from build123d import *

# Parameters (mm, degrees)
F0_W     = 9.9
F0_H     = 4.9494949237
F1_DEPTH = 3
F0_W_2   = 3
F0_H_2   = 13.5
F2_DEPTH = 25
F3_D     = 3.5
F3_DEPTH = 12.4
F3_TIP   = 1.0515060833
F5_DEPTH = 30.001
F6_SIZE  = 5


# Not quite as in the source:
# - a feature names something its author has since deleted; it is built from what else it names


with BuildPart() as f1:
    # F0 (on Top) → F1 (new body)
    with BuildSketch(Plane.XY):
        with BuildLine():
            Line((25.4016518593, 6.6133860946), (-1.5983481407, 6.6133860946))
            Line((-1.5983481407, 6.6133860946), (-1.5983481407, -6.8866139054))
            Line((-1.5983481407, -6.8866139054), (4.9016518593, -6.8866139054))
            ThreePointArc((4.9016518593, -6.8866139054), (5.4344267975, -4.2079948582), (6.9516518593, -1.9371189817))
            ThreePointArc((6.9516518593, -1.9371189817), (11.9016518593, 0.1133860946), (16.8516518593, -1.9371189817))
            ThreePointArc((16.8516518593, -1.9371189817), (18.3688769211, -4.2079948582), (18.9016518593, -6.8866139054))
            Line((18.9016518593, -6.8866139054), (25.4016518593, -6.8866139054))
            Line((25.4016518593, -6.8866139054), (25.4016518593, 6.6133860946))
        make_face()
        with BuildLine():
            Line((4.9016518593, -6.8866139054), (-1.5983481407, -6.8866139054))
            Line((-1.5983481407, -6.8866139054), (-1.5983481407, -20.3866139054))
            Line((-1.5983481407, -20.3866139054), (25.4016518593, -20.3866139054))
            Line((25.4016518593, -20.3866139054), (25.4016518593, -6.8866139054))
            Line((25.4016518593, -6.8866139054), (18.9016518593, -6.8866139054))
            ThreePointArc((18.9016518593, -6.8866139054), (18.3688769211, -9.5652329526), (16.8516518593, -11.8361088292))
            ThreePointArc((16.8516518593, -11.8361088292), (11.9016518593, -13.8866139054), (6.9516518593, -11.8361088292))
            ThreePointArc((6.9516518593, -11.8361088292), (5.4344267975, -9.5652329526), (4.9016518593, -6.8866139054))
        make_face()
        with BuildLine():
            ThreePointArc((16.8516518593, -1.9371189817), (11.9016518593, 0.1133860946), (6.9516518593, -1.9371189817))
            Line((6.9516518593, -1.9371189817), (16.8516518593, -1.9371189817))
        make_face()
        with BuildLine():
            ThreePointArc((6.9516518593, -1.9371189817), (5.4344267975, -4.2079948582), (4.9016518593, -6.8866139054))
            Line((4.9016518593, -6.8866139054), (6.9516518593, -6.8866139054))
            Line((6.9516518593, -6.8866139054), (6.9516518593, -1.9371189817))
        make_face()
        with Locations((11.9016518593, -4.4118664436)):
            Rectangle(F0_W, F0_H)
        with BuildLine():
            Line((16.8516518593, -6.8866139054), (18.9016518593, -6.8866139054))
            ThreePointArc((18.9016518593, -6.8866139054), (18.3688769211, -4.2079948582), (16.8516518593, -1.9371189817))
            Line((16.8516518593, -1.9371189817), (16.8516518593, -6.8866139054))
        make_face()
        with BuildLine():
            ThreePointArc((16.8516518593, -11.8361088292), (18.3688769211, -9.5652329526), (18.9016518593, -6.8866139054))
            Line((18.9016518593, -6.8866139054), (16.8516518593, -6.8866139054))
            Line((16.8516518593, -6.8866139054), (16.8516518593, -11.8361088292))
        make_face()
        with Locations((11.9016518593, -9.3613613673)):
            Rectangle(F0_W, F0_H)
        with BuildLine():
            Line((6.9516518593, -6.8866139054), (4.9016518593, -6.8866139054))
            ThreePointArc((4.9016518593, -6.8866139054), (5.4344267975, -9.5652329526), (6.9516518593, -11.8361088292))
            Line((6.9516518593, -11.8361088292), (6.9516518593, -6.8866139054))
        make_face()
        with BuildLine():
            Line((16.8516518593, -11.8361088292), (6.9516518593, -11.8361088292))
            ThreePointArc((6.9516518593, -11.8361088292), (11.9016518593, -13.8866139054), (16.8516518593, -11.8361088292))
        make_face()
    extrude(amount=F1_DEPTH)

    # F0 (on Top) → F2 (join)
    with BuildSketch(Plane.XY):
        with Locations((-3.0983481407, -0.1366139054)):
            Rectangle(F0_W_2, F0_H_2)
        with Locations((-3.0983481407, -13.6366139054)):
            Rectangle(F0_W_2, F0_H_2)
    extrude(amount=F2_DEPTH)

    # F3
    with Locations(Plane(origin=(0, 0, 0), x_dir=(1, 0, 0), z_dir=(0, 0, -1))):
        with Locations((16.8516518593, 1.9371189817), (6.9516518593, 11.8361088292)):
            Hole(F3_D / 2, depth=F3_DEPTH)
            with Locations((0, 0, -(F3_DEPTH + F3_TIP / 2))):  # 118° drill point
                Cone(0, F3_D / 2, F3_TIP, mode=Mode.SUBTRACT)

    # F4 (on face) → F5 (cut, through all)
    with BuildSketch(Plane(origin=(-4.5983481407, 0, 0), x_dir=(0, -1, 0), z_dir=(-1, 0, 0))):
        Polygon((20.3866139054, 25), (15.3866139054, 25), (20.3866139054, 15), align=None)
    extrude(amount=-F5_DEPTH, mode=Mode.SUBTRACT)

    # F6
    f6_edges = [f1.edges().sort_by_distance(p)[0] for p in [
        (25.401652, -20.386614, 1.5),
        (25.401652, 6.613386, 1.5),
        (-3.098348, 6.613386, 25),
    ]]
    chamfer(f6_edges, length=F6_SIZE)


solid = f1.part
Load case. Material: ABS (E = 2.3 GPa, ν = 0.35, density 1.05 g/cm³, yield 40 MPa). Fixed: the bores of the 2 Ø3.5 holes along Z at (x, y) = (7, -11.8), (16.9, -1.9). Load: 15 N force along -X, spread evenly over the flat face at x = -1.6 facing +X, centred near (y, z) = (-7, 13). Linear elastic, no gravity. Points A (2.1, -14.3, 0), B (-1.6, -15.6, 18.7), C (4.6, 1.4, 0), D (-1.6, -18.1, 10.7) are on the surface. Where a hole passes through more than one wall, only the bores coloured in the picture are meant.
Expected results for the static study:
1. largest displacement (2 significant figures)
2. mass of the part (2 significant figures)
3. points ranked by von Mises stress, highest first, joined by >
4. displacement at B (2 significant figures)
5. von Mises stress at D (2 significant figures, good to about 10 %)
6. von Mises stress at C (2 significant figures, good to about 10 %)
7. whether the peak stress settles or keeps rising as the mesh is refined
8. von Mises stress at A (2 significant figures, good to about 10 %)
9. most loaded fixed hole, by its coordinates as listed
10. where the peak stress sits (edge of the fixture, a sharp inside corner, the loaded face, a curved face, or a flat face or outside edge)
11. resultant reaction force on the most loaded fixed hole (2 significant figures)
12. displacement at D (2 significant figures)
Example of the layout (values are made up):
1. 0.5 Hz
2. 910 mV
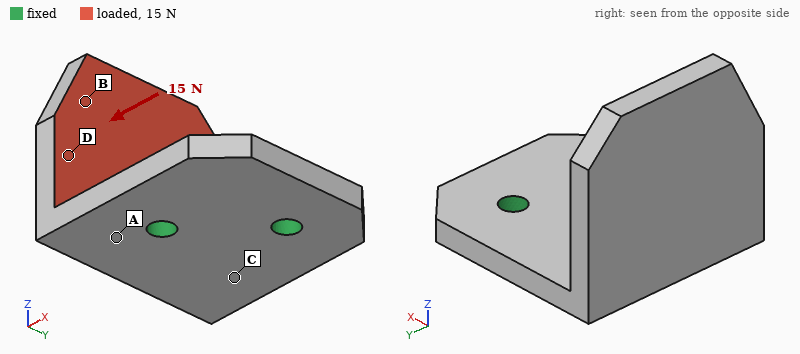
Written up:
1. 0.47 mm
2. 4.2 g
3. A > C > D > B
4. 0.31 mm
5. 1.6 MPa
6. 2.8 MPa
7. keeps rising
8. 4.4 MPa
9. (7, -11.8)
10. edge of the fixture
11. 9.9 N
12. 0.15 mm
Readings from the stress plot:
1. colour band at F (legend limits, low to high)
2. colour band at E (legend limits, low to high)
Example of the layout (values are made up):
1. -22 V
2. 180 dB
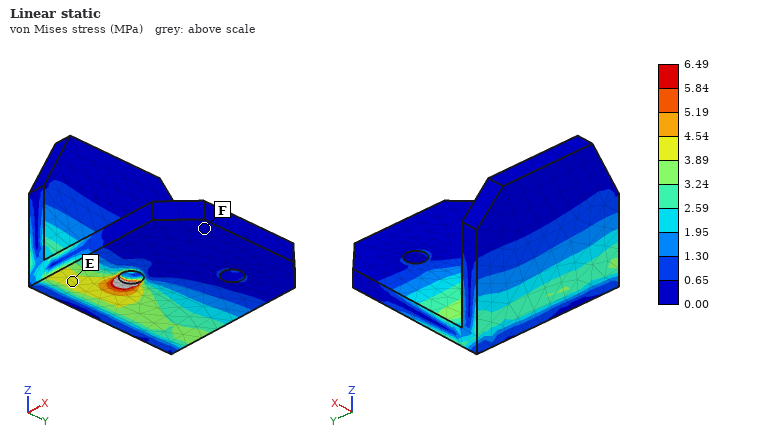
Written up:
1. 0.00 to 0.65 MPa
2. 3.89 to 4.54 MPa
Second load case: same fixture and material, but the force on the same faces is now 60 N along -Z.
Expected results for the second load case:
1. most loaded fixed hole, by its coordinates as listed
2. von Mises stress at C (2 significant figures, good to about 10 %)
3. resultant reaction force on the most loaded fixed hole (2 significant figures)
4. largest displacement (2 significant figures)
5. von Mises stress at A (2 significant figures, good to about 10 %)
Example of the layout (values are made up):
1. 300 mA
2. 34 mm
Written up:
1. (7, -11.8)
2. 4.3 MPa
3. 59 N
4. 0.55 mm
5. 8.4 MPa
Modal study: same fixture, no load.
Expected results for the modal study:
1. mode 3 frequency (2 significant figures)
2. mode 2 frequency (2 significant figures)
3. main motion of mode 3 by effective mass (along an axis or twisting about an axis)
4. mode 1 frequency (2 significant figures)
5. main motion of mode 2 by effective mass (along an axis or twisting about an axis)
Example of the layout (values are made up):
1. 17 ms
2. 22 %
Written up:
1. 2600 Hz
2. 1200 Hz
3. along Z
4. 800 Hz
5. along Y
